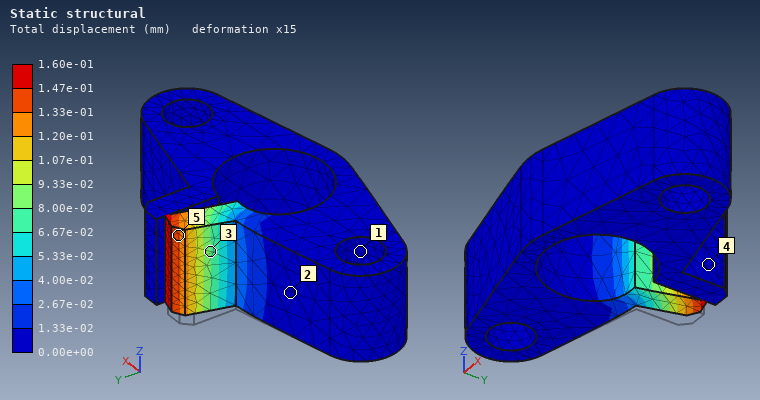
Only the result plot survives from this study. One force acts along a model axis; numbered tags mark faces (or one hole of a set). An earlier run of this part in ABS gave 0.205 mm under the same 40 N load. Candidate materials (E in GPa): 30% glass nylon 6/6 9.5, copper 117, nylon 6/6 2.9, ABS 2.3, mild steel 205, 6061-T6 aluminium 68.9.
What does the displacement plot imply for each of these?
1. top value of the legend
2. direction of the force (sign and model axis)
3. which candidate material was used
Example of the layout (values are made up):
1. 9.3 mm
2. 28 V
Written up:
1. 1.60e-01 mm
2. +X
3. nylon 6/6
